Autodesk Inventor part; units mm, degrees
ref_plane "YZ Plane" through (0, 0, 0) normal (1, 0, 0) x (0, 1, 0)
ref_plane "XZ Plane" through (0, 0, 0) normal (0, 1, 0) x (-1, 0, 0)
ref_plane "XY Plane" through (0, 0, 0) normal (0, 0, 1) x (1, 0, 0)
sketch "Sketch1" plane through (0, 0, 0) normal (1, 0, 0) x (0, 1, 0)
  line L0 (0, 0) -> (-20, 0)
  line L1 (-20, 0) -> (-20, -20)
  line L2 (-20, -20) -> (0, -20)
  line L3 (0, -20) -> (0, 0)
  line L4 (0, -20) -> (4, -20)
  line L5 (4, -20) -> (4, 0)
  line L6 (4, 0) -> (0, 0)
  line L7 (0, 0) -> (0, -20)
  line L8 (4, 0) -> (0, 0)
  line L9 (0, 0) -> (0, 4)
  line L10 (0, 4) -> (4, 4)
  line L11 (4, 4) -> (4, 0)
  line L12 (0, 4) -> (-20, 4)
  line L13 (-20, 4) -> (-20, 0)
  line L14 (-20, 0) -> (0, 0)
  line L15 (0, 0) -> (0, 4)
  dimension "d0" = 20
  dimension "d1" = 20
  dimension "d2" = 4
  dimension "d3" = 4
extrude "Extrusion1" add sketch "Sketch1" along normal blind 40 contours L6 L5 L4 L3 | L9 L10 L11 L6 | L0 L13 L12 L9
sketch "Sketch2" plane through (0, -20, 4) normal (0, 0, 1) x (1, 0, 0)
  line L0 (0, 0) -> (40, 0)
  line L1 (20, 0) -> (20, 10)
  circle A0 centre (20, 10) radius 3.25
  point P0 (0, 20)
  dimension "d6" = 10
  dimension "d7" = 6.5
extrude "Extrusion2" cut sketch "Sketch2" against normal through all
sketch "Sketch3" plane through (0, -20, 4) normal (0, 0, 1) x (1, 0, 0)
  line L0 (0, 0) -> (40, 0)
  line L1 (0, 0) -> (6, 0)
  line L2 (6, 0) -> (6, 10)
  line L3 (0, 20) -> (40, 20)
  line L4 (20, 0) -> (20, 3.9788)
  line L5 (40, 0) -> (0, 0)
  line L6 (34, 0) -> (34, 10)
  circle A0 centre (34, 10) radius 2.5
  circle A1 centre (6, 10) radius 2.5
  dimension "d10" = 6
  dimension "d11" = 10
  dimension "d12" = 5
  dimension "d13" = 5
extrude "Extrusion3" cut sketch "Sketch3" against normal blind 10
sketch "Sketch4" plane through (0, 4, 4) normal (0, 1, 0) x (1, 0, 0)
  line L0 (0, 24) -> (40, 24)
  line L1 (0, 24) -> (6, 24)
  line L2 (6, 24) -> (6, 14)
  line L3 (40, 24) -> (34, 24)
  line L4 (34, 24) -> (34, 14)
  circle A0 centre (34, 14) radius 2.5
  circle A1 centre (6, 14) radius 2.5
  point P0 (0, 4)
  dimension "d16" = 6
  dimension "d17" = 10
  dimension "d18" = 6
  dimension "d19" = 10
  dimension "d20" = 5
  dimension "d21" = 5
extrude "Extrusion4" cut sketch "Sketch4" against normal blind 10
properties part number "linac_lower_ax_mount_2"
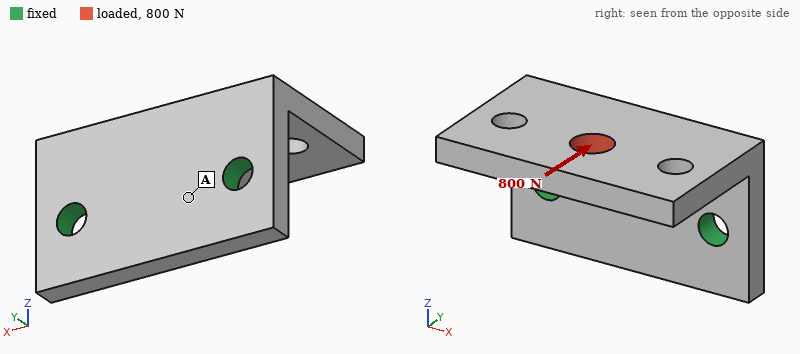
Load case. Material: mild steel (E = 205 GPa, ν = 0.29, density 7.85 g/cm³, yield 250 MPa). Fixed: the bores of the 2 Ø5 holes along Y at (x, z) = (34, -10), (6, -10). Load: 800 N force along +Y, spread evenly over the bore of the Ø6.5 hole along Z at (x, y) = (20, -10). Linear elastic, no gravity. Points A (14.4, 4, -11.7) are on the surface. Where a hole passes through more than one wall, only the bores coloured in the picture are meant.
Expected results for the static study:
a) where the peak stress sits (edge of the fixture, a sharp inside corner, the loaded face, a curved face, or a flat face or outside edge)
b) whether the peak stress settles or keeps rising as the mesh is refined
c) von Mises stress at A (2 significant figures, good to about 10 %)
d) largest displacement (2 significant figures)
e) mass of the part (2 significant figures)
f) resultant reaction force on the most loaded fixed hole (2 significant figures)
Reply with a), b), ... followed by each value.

a) edge of the fixture
b) keeps rising
c) 19 MPa
d) 30 µm
e) 52 g
f) 400 N
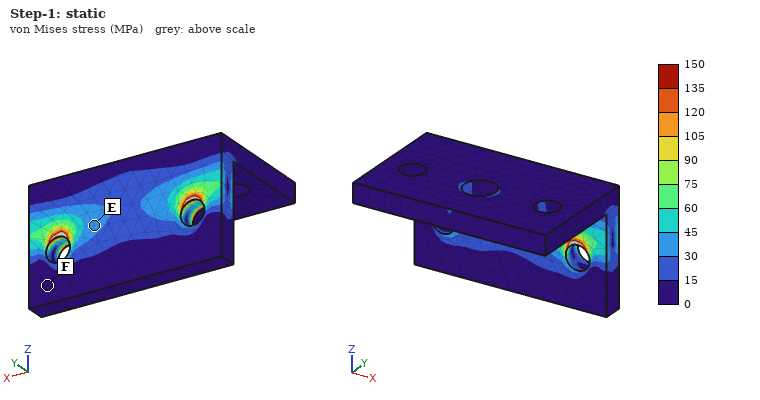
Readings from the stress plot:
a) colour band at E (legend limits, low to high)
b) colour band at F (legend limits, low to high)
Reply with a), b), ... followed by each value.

a) 30 to 45 MPa
b) 0 to 15 MPa
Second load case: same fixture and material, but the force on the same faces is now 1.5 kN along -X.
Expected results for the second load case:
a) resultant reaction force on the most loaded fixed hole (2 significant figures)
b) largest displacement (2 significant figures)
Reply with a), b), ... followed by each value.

a) 1.1 kN
b) 26 µm
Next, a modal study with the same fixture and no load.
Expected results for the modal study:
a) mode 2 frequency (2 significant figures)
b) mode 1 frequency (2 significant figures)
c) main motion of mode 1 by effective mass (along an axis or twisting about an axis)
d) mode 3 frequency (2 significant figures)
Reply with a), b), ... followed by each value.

a) 7300 Hz
b) 3900 Hz
c) along Z
d) 11 kHz
